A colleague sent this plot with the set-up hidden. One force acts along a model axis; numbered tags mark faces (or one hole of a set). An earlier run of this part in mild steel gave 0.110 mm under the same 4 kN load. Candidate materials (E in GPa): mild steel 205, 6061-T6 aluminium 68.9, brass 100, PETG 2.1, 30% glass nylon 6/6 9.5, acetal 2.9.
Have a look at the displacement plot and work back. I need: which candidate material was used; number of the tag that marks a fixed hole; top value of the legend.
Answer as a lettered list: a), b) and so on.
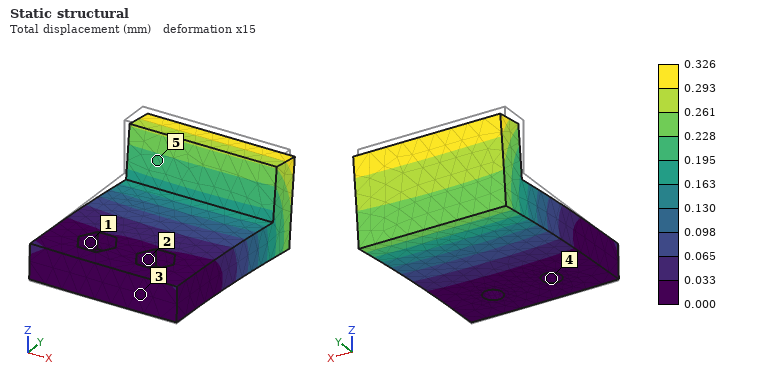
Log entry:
a) 6061-T6 aluminium
b) 4
c) 0.326 mm
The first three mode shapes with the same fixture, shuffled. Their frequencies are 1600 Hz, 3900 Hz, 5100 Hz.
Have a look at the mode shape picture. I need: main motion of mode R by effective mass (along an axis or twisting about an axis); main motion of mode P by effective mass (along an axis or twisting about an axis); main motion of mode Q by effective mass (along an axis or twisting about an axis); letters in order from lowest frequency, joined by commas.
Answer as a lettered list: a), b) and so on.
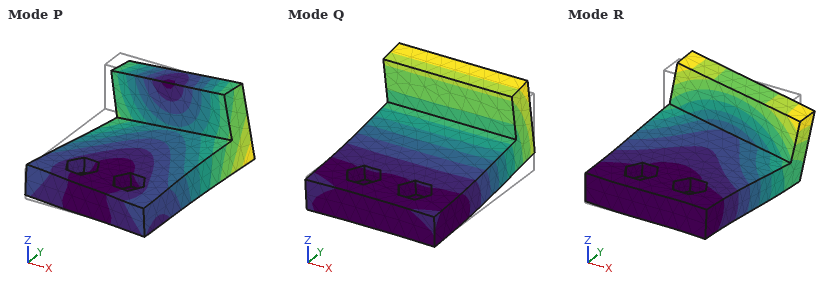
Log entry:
a) along X
b) along X
c) along Z
d) Q, R, P
